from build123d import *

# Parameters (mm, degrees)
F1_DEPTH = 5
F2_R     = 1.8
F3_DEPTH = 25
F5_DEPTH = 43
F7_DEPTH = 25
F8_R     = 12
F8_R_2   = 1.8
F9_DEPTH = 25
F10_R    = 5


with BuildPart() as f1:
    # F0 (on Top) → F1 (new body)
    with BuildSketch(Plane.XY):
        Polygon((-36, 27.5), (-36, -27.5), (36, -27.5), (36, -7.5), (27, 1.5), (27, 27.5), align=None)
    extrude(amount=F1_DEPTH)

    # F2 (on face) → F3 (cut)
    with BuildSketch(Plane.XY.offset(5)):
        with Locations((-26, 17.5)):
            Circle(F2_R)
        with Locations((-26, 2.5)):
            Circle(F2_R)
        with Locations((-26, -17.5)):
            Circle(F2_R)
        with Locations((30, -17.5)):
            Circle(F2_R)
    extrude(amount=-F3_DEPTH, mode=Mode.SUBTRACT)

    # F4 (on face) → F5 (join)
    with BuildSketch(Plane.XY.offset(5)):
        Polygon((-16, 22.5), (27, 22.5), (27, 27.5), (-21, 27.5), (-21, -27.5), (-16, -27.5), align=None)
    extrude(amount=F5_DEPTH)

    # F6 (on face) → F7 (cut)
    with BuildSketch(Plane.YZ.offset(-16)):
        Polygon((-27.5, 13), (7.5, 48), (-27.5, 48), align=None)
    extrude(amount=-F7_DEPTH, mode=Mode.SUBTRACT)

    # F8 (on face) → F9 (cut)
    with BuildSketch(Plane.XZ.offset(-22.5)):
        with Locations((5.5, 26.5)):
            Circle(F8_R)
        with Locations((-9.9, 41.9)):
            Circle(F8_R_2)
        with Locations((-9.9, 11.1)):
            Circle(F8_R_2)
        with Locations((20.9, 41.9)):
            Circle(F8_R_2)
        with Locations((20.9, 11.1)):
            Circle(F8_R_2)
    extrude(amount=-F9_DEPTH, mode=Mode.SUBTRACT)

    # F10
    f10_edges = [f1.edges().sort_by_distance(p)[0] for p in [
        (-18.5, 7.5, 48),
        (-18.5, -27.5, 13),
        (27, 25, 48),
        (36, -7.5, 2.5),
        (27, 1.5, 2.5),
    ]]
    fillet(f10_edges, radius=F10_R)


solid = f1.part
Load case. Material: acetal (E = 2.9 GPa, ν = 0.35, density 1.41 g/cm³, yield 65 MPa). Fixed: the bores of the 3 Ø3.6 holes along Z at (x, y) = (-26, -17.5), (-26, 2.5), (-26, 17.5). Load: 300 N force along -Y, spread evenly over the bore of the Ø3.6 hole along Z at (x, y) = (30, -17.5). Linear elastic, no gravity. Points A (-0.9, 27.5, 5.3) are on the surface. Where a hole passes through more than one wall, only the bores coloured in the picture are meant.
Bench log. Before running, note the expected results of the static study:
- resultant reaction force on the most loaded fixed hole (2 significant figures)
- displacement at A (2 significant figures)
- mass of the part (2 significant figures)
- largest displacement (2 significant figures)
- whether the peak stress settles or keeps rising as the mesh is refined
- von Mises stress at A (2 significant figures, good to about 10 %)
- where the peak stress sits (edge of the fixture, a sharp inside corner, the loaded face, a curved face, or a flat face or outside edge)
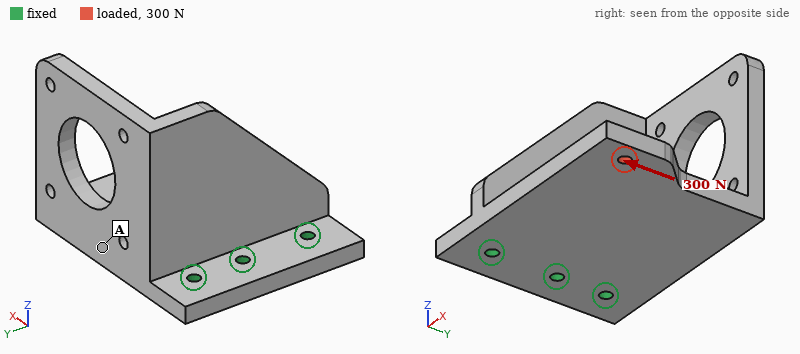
470 N
0.090 mm
48 g
0.26 mm
keeps rising
1.7 MPa
edge of the fixture
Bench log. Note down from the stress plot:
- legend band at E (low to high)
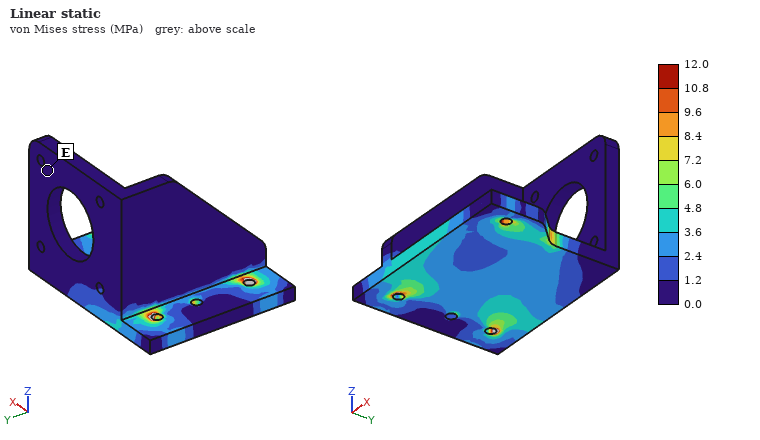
0.0 to 1.2 MPa
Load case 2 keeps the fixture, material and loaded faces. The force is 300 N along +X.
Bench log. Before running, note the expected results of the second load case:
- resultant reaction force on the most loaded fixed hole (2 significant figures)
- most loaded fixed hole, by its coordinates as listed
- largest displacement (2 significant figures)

260 N
(-26, -17.5)
89 µm
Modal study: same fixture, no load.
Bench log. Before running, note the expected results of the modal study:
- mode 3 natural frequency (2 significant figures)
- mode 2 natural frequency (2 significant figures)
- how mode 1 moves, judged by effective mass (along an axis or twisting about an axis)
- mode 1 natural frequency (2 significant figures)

840 Hz
630 Hz
along Z
300 Hz
